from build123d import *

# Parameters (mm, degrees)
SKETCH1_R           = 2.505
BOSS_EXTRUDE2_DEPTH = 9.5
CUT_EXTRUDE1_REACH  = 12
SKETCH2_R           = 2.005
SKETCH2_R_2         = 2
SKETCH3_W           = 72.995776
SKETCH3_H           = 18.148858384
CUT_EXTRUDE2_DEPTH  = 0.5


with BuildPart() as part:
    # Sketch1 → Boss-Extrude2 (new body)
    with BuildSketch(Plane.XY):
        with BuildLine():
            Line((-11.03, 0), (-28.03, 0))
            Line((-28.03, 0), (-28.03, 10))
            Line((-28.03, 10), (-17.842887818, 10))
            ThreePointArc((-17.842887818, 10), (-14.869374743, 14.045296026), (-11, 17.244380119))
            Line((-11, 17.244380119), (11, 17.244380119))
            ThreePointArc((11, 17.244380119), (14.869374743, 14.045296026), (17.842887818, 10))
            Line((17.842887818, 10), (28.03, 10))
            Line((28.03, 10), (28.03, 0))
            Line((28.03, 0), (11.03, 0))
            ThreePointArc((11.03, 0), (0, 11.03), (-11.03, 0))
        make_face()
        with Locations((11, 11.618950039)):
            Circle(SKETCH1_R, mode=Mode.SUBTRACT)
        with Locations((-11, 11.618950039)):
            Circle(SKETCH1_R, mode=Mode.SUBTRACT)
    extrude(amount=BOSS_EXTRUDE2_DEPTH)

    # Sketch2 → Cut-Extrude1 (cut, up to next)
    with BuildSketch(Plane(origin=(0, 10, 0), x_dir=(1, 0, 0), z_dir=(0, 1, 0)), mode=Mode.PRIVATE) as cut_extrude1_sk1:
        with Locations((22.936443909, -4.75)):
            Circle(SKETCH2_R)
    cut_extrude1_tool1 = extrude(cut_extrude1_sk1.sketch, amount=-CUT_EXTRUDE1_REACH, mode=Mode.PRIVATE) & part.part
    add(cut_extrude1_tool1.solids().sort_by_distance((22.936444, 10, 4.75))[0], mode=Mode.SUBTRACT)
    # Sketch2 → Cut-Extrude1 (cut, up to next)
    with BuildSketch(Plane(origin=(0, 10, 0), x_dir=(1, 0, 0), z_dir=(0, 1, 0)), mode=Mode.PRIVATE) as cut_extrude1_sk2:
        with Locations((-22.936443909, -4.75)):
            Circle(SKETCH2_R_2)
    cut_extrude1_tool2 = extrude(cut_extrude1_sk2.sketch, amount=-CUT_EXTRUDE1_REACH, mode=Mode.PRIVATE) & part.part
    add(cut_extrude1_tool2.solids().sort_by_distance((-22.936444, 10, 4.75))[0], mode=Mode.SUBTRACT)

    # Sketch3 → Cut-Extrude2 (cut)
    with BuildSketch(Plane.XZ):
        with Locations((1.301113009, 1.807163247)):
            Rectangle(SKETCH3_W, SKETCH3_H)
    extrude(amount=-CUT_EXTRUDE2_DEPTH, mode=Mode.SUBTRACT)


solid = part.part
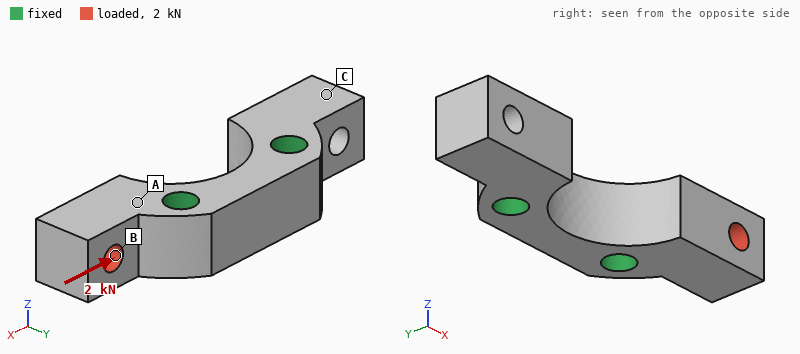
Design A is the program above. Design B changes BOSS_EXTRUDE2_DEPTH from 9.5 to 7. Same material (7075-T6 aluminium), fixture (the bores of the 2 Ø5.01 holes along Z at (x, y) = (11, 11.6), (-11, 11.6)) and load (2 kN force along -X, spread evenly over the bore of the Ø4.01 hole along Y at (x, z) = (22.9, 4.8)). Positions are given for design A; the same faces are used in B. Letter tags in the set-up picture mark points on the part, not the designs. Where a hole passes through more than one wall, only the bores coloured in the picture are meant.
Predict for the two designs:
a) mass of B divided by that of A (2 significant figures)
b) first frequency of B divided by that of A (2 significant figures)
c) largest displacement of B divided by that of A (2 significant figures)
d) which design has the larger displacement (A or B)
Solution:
0.72
0.90
1.9
B
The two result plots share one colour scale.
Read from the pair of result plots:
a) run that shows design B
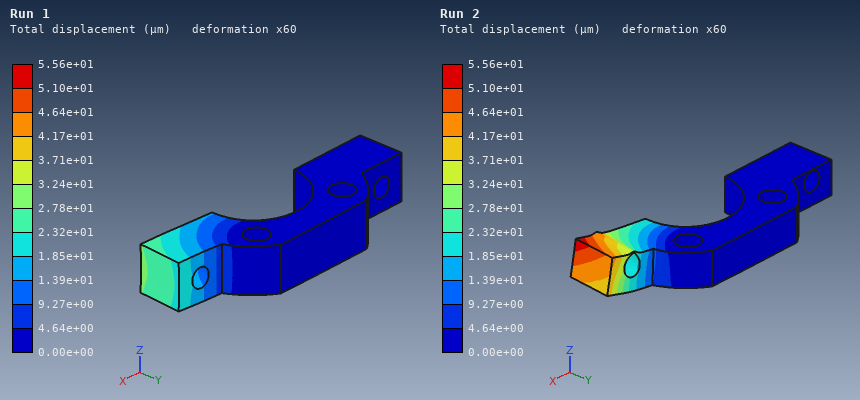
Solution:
Run 2
